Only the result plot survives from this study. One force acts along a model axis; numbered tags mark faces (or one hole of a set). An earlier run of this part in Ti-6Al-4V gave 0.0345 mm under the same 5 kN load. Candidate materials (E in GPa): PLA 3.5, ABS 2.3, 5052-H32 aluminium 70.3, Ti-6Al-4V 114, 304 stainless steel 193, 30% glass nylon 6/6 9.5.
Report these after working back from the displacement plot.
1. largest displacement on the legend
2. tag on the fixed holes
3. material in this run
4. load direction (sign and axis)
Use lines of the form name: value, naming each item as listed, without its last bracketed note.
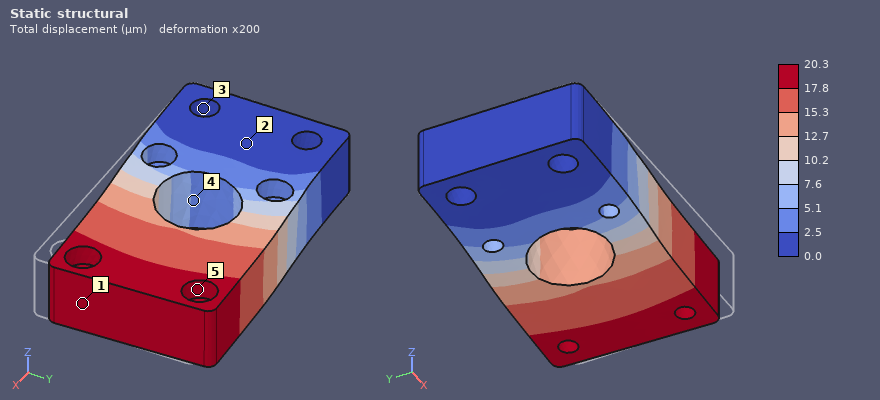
largest displacement on the legend: 20.3 µm
tag on the fixed holes: 3
material in this run: 304 stainless steel
load direction: +Y
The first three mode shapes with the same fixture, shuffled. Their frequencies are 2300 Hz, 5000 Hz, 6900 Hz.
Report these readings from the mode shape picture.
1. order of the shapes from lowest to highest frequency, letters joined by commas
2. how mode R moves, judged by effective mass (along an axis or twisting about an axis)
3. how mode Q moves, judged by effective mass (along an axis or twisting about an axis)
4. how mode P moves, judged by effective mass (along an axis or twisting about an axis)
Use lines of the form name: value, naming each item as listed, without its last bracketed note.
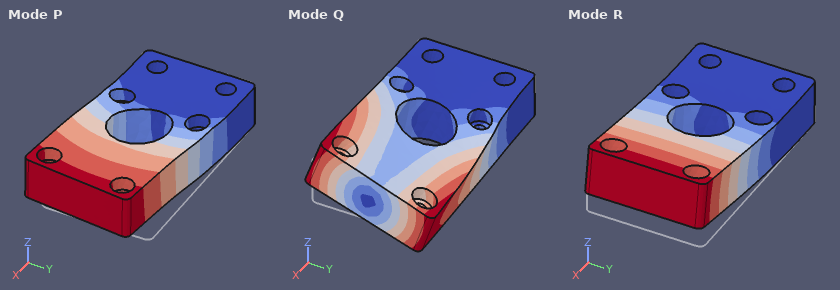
order of the shapes from lowest to highest frequency, letters joined by commas: R, P, Q
how mode R moves, judged by effective mass: along Z
how mode Q moves, judged by effective mass: twisting about X
how mode P moves, judged by effective mass: along Y
